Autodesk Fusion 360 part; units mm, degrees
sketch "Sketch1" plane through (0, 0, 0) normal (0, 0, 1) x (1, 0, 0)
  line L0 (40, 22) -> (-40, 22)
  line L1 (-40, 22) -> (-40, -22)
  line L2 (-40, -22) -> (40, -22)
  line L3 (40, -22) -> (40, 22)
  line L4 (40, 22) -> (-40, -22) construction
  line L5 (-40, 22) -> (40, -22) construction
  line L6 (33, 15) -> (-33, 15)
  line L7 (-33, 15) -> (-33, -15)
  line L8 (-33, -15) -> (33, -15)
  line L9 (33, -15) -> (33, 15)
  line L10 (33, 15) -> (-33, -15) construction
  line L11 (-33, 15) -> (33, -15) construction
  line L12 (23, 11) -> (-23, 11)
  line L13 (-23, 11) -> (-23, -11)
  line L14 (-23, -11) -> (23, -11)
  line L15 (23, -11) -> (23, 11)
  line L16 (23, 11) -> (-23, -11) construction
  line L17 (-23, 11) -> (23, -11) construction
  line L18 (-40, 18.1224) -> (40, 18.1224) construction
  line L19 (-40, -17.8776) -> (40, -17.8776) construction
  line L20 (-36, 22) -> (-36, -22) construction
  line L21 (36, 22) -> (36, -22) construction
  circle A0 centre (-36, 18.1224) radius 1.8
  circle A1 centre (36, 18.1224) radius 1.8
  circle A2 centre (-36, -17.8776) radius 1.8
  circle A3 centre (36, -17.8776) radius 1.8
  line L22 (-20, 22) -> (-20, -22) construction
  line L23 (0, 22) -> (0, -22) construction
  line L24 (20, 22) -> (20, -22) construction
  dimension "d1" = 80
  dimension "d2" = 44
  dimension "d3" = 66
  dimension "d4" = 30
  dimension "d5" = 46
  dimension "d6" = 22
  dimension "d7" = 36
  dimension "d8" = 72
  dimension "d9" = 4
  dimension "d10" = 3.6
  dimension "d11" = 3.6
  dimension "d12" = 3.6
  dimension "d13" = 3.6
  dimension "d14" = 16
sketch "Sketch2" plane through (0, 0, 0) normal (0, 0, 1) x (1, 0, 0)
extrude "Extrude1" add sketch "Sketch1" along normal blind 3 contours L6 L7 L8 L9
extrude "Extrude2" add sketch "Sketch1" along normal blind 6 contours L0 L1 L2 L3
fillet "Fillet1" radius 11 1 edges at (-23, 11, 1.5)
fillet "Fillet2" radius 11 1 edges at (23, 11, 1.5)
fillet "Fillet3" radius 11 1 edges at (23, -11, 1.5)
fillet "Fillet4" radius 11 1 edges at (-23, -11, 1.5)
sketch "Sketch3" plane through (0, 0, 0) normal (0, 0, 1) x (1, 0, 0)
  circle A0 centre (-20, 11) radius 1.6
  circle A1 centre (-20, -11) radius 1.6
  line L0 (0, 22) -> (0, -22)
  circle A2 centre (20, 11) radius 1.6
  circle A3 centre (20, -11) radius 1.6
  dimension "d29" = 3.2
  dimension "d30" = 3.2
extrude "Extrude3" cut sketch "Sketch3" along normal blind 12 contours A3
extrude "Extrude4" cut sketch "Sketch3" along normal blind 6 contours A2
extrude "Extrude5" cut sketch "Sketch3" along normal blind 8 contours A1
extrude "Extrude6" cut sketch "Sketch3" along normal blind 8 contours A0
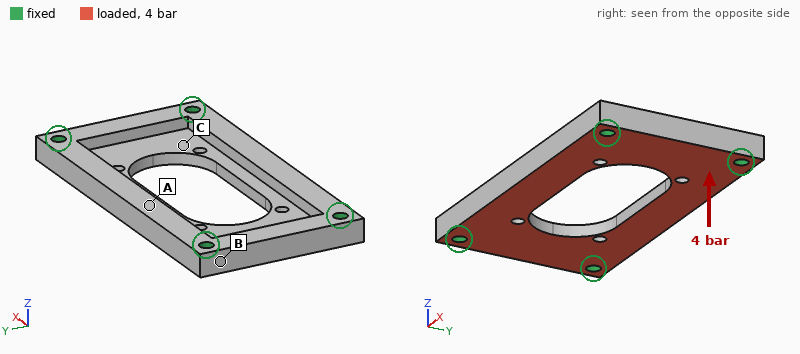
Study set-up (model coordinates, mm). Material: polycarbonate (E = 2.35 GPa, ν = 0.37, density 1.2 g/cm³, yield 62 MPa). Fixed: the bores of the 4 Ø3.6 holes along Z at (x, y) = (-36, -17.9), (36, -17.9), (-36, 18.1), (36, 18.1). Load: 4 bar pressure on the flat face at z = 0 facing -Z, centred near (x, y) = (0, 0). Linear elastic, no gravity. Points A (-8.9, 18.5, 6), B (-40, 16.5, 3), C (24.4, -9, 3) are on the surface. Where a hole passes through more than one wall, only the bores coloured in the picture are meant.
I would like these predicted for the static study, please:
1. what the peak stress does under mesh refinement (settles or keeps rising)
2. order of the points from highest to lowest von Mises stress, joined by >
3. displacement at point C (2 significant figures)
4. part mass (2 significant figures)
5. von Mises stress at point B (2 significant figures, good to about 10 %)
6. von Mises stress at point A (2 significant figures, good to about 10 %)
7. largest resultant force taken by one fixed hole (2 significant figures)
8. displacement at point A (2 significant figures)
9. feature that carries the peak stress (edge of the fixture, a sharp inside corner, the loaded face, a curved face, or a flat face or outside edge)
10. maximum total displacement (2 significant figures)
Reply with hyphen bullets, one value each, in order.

- keeps rising
- A > B > C
- 0.38 mm
- 15 g
- 9.6 MPa
- 16 MPa
- 260 N
- 0.79 mm
- edge of the fixture
- 1.1 mm
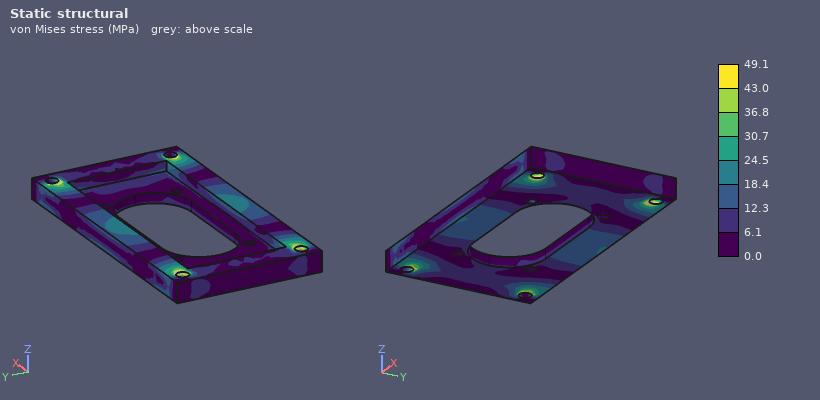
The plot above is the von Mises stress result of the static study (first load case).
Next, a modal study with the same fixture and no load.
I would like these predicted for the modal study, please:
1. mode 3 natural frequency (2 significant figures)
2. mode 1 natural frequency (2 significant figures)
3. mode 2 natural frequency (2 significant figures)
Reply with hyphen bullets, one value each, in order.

- 3300 Hz
- 1600 Hz
- 1700 Hz
